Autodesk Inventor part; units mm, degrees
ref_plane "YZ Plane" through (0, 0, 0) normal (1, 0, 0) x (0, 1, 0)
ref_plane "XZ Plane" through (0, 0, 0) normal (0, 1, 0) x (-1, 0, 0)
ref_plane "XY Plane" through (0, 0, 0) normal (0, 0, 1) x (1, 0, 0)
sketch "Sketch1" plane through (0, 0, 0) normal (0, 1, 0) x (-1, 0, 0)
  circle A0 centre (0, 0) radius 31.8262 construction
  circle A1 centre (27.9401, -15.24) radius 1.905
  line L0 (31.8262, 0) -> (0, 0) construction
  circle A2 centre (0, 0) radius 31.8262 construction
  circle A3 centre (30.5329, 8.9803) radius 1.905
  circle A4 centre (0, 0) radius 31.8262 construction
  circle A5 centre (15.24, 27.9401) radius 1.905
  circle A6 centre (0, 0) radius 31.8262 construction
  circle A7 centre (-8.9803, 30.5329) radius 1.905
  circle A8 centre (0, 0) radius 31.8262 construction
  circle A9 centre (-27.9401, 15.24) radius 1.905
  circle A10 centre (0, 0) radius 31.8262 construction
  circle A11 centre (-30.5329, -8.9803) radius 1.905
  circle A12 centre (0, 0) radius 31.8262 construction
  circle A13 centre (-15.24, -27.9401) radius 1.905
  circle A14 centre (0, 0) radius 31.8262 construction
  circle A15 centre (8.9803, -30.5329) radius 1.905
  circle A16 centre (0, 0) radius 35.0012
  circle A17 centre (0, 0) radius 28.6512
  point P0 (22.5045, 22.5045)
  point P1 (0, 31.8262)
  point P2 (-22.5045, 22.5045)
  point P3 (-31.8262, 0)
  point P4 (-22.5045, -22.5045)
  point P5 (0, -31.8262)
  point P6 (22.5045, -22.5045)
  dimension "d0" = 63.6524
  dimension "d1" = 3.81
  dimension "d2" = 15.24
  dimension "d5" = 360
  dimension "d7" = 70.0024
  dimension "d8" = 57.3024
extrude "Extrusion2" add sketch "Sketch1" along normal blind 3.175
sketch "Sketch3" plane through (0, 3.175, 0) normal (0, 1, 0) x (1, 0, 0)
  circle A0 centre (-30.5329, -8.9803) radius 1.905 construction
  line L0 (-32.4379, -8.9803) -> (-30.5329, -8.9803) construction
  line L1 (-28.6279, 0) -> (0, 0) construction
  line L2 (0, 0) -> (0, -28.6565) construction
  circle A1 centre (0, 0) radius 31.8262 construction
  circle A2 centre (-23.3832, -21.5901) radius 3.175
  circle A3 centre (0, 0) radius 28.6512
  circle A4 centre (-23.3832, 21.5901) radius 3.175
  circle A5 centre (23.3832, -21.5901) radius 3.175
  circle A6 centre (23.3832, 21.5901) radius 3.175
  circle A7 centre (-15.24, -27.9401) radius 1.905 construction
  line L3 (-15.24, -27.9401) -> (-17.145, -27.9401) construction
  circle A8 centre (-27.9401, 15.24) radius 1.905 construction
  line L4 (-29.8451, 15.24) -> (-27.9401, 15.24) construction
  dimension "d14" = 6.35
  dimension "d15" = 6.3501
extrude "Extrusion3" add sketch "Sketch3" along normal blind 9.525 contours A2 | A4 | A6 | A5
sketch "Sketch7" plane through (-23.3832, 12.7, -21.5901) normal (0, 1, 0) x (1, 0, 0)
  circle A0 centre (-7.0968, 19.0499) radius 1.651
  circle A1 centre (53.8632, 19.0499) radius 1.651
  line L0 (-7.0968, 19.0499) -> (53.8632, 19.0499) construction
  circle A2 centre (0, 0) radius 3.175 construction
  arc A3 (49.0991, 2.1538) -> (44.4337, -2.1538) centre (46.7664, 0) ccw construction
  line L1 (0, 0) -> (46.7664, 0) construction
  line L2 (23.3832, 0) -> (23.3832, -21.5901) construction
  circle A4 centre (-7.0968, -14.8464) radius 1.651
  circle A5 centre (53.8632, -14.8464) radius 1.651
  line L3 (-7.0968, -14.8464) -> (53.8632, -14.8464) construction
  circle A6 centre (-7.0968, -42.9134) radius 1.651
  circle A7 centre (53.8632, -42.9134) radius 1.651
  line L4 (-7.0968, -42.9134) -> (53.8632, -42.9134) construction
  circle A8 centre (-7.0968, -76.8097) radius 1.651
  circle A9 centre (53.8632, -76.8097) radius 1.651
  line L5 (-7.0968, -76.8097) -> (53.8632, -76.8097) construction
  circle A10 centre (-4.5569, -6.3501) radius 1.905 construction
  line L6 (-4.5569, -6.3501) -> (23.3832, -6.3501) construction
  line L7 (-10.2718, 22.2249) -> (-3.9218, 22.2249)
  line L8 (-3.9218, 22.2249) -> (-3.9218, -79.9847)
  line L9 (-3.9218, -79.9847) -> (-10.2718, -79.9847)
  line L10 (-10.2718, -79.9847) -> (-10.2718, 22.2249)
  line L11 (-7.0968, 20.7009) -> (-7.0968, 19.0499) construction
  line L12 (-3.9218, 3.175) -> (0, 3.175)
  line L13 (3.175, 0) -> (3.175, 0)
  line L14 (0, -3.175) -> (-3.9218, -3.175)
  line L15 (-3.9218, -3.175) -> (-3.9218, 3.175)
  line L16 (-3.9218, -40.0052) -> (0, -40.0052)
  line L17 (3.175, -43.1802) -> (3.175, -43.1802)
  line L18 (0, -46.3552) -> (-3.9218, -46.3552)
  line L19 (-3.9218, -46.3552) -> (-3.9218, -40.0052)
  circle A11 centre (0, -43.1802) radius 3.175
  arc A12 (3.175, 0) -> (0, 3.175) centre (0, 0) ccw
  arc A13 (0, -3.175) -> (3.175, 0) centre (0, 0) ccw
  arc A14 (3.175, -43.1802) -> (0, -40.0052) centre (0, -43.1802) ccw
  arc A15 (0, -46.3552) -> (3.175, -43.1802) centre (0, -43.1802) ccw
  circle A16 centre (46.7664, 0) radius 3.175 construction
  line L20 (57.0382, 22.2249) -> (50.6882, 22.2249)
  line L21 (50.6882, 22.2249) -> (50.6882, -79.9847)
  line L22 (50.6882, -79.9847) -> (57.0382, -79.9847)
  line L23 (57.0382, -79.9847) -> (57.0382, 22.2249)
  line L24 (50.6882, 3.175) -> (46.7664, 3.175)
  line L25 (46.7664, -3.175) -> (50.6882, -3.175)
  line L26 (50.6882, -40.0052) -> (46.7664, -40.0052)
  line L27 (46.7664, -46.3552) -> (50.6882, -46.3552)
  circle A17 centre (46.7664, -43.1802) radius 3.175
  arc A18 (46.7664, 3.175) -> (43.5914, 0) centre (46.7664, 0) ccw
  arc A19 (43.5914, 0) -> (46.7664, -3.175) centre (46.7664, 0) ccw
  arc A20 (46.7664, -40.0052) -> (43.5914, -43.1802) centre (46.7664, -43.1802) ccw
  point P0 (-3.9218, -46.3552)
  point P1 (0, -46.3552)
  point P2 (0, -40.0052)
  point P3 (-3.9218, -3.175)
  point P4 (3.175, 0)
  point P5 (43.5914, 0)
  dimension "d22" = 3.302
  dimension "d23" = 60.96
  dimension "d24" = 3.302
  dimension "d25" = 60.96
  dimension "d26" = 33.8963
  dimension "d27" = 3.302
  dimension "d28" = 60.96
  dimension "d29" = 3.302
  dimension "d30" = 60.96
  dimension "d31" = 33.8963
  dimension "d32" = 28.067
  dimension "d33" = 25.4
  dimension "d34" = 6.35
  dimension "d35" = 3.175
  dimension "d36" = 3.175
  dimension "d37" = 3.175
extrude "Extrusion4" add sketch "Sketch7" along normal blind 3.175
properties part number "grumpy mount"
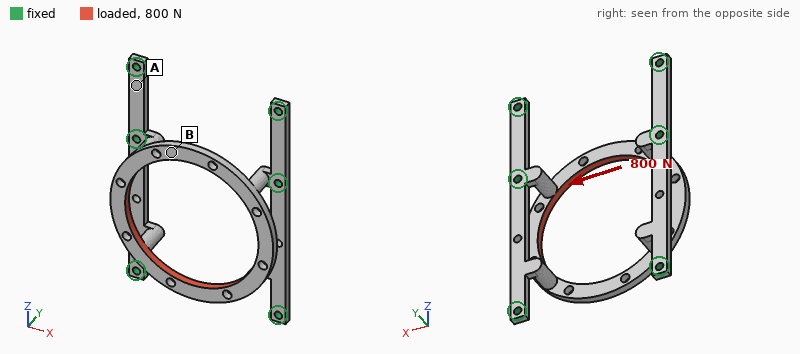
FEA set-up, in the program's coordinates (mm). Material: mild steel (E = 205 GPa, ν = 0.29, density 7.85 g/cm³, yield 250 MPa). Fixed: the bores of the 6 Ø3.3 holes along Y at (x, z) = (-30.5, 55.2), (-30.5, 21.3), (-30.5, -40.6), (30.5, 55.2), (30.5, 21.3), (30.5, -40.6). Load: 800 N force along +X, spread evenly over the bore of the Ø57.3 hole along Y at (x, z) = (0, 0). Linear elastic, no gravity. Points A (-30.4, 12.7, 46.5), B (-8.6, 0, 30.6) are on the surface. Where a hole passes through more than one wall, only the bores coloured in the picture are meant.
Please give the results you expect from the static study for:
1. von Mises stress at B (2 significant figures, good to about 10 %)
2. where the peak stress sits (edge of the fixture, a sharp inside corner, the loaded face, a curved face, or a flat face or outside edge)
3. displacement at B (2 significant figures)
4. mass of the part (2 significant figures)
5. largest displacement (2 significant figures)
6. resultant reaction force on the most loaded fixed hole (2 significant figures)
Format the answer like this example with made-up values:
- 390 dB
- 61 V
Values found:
- 30 MPa
- a curved face
- 31 µm
- 74 g
- 59 µm
- 270 N
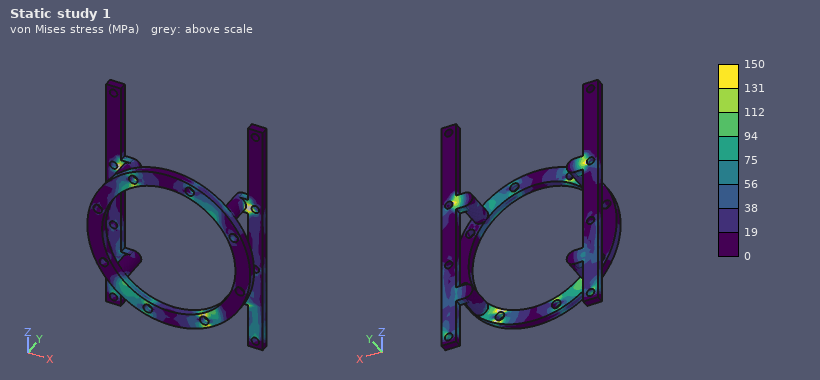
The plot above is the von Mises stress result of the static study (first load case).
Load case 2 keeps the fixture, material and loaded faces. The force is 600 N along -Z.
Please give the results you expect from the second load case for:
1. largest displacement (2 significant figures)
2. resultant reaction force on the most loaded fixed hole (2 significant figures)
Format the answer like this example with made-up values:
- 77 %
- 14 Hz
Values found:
- 40 µm
- 200 N
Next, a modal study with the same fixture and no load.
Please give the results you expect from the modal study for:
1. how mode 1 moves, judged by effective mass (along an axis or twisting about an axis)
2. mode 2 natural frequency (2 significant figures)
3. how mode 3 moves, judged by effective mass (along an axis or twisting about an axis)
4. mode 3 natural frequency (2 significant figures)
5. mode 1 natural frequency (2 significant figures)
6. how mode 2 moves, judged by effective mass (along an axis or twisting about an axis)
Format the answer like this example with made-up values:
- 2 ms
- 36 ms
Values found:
- along Y
- 3400 Hz
- twisting about Z
- 3600 Hz
- 3100 Hz
- along X
